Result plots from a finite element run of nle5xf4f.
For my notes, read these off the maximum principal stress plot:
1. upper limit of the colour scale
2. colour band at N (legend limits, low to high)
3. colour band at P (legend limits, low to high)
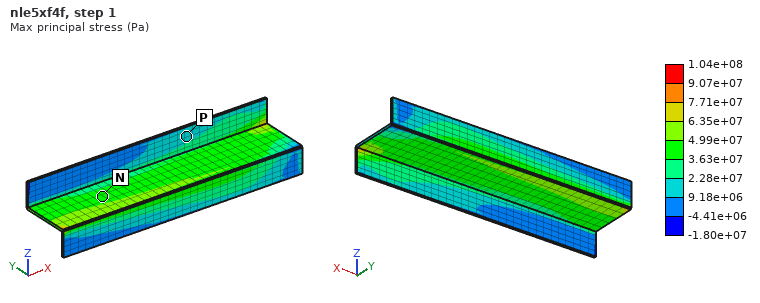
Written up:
1.04e+08 Pa
3.63e+07 to 4.99e+07 Pa
9.18e+06 to 2.28e+07 Pa
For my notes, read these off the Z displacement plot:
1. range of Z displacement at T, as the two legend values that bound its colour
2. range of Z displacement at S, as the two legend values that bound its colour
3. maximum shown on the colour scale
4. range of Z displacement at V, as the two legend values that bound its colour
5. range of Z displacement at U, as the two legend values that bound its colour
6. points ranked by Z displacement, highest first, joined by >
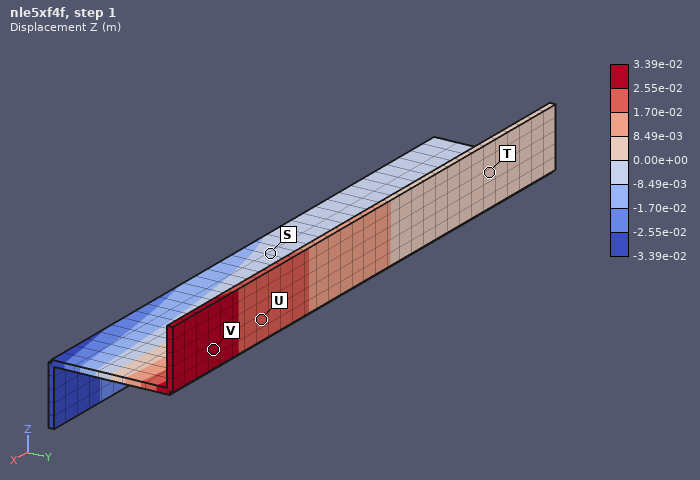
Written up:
0.00e+00 to 8.49e-03 m
-8.49e-03 to 0.00e+00 m
3.39e-02 m
2.55e-02 to 3.39e-02 m
1.70e-02 to 2.55e-02 m
V > U > T > S
